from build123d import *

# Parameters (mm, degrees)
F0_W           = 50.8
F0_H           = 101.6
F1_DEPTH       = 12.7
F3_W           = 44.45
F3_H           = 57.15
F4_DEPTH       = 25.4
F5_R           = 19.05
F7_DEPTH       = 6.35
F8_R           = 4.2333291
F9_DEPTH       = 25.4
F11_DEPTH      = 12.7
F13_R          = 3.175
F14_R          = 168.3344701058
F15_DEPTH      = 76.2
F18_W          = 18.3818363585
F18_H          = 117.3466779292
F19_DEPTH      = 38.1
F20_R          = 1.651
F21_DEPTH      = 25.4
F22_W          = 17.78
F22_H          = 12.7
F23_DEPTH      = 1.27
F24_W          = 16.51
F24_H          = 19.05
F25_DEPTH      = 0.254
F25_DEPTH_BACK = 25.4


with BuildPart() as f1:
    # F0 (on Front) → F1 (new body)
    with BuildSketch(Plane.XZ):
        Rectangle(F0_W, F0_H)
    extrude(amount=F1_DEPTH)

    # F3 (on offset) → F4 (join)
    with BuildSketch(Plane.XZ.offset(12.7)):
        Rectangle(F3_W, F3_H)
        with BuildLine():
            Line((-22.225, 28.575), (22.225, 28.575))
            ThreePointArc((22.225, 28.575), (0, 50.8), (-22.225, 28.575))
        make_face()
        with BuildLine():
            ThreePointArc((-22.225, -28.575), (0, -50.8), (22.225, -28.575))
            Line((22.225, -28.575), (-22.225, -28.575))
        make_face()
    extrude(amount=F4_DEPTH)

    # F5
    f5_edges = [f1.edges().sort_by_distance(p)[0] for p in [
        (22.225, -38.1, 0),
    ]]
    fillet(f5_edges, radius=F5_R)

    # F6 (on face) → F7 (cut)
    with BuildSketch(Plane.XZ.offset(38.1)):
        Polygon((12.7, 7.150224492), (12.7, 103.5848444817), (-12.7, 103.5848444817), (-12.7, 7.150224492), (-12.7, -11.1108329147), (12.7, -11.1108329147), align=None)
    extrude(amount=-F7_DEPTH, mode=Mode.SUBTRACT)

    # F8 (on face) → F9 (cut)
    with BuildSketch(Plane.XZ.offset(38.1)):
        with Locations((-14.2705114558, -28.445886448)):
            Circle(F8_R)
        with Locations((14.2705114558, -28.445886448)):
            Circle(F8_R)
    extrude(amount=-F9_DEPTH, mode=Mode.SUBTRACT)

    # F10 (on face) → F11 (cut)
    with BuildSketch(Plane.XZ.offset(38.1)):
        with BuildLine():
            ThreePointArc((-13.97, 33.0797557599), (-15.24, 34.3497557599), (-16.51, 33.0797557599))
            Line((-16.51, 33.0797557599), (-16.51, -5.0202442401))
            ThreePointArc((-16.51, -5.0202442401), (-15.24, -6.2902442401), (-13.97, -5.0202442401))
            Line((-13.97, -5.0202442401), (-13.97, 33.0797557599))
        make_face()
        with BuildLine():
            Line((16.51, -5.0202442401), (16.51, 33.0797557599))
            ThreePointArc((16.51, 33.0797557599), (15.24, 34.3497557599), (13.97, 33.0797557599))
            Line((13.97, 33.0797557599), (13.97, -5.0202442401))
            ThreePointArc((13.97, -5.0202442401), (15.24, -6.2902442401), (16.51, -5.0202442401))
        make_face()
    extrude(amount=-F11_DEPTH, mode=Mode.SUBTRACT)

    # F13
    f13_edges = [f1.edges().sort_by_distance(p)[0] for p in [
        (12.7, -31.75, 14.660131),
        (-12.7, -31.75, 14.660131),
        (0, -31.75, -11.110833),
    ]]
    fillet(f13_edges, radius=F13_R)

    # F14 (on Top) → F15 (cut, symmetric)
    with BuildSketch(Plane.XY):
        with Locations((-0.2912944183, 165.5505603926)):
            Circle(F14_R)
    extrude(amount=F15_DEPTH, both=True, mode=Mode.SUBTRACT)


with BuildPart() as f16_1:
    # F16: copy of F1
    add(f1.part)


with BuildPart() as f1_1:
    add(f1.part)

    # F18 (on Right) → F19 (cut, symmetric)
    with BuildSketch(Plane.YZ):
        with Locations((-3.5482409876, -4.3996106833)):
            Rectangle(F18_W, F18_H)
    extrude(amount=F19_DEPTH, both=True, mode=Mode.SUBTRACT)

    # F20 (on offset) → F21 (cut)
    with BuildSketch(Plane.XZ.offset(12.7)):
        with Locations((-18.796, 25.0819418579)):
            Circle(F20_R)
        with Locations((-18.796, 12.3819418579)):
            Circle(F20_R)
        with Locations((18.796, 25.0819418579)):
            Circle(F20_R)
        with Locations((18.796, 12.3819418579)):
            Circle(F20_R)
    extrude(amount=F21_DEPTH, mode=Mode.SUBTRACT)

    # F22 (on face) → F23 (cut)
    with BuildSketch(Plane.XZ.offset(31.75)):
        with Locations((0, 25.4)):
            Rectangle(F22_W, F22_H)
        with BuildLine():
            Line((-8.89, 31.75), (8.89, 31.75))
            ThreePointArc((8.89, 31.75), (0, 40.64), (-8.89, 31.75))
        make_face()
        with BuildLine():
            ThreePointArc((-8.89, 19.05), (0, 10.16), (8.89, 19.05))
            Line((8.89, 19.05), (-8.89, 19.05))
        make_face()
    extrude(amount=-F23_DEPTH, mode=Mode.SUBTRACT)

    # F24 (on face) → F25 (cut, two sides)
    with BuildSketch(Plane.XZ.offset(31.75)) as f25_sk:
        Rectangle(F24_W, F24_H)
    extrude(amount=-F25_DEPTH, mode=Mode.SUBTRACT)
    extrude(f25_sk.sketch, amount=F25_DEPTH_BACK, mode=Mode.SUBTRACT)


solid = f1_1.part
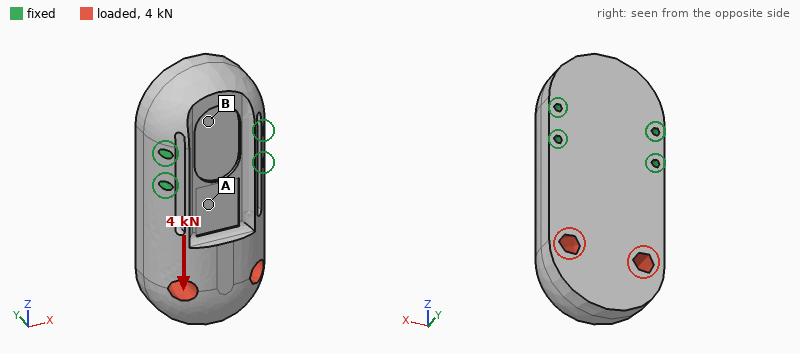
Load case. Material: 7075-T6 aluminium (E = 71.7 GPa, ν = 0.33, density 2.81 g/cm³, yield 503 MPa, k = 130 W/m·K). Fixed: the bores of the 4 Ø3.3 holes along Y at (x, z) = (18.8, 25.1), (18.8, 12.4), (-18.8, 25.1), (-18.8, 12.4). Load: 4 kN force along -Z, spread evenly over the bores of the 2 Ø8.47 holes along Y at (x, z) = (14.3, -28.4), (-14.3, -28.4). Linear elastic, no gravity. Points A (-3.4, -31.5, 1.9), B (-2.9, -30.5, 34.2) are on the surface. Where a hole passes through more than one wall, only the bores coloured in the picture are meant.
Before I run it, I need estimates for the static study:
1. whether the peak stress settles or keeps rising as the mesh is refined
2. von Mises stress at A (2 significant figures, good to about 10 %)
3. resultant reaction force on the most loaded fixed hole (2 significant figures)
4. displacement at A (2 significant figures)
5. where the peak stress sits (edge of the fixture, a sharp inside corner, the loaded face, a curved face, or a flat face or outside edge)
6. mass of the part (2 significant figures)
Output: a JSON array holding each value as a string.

["keeps rising", "5.5 MPa", "1.4 kN", "3.2 µm", "edge of the fixture", "210 g"]
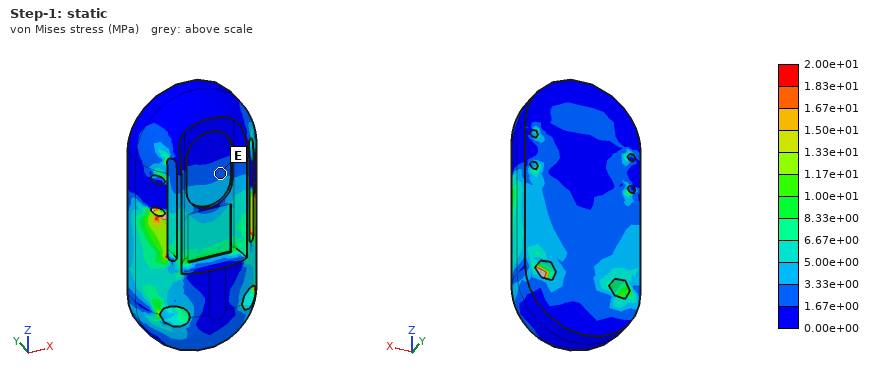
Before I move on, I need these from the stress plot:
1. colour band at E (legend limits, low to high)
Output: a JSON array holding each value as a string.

["1.67e+00 to 3.33e+00 MPa"]
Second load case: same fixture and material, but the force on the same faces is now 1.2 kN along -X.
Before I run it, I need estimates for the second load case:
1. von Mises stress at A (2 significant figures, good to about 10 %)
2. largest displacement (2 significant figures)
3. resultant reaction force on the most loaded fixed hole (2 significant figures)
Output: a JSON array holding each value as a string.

["3.0 MPa", "9.2 µm", "1.3 kN"]
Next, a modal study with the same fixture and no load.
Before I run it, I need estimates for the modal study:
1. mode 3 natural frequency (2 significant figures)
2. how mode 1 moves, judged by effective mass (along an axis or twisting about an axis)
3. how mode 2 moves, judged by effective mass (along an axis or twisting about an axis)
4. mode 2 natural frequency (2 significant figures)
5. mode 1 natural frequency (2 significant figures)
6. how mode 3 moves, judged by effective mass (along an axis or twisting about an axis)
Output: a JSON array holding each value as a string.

["10 kHz", "along Y", "along X", "7200 Hz", "3300 Hz", "twisting about Z"]
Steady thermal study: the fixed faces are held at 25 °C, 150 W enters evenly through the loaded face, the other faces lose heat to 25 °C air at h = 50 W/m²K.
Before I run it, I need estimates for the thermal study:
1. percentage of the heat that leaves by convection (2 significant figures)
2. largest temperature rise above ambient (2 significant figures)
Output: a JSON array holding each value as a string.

["12 %", "68 K"]
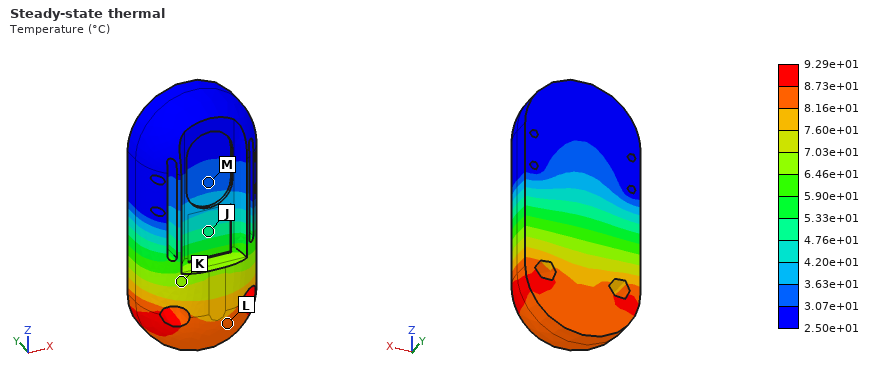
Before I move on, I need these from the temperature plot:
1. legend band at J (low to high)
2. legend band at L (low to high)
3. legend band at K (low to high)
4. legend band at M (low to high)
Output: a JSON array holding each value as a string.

["4.76e+01 to 5.33e+01 °C", "8.16e+01 to 8.73e+01 °C", "6.46e+01 to 7.03e+01 °C", "3.07e+01 to 3.63e+01 °C"]
